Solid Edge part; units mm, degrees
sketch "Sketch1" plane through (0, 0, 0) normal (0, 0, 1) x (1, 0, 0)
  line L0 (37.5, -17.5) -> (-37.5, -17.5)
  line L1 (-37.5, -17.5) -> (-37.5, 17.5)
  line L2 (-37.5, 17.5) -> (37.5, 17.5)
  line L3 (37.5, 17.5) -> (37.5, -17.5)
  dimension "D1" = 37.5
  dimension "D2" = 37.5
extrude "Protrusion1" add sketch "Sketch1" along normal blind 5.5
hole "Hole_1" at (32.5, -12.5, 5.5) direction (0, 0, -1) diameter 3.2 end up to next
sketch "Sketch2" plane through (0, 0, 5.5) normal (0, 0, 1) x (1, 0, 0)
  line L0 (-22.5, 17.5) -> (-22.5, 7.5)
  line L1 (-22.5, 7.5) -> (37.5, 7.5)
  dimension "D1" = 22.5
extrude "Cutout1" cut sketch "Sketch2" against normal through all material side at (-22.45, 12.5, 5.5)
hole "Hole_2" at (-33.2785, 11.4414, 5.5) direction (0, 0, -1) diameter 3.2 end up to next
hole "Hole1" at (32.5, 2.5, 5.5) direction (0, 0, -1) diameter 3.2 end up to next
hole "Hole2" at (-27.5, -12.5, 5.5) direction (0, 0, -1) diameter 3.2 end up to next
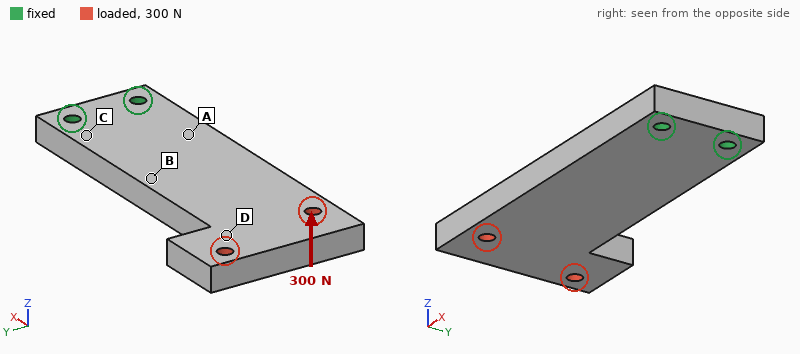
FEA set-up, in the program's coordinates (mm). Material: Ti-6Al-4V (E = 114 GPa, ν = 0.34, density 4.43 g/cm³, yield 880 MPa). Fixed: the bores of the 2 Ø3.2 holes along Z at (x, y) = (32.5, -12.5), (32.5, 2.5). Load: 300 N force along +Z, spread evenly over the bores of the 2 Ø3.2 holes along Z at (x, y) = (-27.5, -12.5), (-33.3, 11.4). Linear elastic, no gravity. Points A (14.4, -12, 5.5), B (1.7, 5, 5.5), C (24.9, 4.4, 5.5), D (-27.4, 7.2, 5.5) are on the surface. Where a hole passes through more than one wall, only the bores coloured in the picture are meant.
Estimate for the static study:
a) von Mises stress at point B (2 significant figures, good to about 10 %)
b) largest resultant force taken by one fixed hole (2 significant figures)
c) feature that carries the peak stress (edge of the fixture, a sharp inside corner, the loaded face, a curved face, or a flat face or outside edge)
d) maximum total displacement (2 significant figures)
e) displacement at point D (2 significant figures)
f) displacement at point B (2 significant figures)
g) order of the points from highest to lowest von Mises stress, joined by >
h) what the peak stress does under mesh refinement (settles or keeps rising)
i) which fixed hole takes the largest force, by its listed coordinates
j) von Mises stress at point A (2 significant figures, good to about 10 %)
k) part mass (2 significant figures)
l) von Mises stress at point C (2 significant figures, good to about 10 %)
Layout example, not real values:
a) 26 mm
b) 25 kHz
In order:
a) 77 MPa
b) 220 N
c) edge of the fixture
d) 0.78 mm
e) 0.60 mm
f) 0.20 mm
g) C > A > B > D
h) keeps rising
i) (32.5, 2.5)
j) 100 MPa
k) 49 g
l) 140 MPa
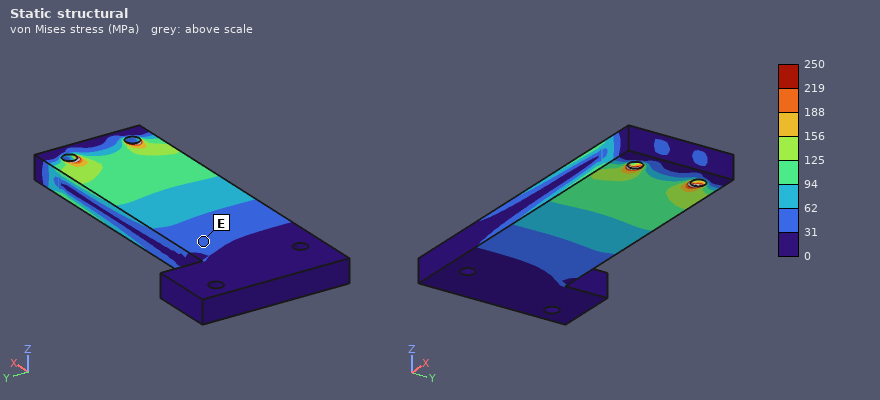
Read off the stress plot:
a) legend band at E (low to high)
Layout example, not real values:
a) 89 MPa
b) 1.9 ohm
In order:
a) 31 to 62 MPa
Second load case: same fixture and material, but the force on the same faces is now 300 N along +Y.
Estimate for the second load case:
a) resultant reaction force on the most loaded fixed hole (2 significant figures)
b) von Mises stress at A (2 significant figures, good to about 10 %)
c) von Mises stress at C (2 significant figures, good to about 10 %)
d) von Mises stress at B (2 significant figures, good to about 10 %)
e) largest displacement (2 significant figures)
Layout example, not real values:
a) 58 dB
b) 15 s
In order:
a) 1.1 kN
b) 14 MPa
c) 22 MPa
d) 14 MPa
e) 46 µm
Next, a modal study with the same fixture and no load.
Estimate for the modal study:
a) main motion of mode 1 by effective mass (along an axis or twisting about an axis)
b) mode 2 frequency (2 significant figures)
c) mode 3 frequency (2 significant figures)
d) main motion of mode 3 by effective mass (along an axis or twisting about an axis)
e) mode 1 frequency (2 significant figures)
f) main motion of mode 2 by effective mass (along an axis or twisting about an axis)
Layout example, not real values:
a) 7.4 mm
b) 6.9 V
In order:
a) along Z
b) 3300 Hz
c) 3500 Hz
d) twisting about X
e) 830 Hz
f) along Y
